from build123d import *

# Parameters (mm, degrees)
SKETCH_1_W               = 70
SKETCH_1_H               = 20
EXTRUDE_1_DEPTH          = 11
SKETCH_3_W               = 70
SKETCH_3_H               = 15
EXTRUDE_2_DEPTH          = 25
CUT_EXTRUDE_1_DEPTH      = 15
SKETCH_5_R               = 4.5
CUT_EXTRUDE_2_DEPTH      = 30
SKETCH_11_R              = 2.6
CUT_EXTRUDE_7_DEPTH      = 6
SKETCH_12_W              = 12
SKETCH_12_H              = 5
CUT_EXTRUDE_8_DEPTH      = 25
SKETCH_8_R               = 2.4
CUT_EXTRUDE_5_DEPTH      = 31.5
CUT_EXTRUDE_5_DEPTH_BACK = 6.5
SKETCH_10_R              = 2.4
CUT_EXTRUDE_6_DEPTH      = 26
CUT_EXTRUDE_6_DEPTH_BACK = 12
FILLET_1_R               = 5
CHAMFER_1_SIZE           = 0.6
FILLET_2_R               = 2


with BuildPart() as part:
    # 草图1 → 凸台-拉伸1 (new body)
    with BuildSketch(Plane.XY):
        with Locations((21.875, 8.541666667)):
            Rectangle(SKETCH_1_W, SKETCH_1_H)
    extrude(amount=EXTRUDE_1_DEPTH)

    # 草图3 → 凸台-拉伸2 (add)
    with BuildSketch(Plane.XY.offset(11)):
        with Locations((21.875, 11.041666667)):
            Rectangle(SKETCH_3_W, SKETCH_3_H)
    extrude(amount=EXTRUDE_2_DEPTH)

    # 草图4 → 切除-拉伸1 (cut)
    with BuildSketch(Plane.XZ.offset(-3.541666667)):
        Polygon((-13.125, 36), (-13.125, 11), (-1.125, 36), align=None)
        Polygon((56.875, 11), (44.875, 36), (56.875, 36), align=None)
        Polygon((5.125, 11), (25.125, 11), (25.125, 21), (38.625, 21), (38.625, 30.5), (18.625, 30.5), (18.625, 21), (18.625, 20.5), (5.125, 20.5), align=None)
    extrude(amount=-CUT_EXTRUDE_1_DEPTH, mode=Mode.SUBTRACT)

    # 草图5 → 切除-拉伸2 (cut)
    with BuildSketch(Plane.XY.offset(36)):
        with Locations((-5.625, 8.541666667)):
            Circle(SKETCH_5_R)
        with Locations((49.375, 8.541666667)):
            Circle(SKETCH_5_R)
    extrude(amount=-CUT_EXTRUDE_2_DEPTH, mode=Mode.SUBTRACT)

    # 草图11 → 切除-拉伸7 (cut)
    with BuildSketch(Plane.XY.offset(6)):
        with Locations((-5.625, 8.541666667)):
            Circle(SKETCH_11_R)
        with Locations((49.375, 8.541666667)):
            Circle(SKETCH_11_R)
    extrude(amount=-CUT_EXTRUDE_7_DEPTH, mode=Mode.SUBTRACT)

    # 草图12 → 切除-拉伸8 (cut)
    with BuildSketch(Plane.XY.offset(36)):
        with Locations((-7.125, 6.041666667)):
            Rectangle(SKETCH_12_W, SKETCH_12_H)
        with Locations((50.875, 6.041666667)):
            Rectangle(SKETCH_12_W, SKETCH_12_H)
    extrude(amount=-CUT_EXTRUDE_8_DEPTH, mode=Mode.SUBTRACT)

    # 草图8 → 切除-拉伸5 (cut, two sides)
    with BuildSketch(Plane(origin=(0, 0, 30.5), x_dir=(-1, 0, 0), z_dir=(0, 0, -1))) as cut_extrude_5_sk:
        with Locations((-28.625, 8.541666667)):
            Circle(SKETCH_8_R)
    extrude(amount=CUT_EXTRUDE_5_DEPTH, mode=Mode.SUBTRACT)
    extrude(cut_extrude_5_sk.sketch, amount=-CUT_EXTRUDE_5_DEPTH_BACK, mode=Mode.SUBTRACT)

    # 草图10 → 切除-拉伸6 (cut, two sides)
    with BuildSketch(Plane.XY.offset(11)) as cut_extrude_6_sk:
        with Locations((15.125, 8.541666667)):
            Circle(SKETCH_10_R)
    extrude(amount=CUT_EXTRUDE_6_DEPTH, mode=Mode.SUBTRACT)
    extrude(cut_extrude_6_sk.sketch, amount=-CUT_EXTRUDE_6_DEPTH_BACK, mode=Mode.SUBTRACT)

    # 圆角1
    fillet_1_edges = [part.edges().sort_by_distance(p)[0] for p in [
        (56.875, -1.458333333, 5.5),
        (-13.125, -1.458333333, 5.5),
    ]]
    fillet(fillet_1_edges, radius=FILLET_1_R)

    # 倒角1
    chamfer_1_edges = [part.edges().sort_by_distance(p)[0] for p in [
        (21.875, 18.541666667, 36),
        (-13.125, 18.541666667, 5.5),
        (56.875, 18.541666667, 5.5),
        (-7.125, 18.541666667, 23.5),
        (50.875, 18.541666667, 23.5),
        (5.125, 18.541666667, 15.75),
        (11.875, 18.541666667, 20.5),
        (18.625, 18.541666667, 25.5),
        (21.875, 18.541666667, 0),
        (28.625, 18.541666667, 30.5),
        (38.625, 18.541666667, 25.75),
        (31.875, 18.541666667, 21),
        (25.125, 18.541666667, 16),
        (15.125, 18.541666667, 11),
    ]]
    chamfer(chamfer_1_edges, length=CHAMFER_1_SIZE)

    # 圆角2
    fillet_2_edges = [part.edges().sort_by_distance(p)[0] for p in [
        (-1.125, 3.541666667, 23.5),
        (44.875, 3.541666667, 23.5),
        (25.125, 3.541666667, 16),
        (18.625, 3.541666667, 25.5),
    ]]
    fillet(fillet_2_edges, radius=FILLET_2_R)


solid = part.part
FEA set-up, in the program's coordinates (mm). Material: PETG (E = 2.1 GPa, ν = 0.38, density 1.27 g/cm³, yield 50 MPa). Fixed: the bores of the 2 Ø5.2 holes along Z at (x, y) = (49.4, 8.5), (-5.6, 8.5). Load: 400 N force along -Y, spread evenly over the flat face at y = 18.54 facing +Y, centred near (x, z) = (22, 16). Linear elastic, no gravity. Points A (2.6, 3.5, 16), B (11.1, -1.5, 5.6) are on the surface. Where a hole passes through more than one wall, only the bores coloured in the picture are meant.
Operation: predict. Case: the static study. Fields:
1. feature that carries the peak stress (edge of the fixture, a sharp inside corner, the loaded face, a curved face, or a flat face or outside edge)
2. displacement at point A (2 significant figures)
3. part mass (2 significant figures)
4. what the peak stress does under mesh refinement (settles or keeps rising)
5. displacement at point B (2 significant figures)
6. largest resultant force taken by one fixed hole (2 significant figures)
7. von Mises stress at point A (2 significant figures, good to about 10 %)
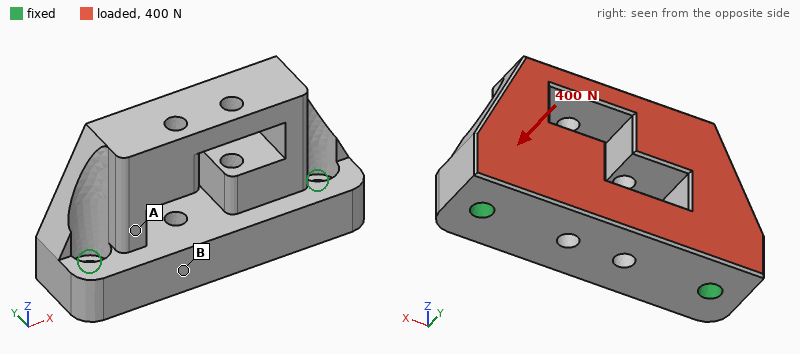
edge of the fixture
0.15 mm
34 g
keeps rising
0.10 mm
200 N
3.3 MPa
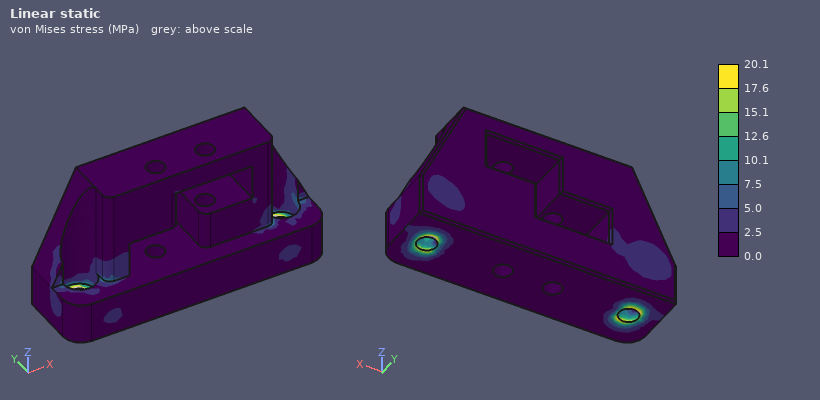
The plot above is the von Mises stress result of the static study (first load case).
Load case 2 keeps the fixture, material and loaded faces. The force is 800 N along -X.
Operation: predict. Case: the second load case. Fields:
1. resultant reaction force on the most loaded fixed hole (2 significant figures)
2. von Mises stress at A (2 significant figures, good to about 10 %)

460 N
1.8 MPa
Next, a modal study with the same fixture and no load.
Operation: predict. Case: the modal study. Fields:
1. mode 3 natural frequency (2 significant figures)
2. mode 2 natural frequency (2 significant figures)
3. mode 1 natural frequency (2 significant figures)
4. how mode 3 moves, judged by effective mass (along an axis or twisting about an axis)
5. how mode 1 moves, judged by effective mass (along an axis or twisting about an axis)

2500 Hz
2400 Hz
1100 Hz
along X
along Y
